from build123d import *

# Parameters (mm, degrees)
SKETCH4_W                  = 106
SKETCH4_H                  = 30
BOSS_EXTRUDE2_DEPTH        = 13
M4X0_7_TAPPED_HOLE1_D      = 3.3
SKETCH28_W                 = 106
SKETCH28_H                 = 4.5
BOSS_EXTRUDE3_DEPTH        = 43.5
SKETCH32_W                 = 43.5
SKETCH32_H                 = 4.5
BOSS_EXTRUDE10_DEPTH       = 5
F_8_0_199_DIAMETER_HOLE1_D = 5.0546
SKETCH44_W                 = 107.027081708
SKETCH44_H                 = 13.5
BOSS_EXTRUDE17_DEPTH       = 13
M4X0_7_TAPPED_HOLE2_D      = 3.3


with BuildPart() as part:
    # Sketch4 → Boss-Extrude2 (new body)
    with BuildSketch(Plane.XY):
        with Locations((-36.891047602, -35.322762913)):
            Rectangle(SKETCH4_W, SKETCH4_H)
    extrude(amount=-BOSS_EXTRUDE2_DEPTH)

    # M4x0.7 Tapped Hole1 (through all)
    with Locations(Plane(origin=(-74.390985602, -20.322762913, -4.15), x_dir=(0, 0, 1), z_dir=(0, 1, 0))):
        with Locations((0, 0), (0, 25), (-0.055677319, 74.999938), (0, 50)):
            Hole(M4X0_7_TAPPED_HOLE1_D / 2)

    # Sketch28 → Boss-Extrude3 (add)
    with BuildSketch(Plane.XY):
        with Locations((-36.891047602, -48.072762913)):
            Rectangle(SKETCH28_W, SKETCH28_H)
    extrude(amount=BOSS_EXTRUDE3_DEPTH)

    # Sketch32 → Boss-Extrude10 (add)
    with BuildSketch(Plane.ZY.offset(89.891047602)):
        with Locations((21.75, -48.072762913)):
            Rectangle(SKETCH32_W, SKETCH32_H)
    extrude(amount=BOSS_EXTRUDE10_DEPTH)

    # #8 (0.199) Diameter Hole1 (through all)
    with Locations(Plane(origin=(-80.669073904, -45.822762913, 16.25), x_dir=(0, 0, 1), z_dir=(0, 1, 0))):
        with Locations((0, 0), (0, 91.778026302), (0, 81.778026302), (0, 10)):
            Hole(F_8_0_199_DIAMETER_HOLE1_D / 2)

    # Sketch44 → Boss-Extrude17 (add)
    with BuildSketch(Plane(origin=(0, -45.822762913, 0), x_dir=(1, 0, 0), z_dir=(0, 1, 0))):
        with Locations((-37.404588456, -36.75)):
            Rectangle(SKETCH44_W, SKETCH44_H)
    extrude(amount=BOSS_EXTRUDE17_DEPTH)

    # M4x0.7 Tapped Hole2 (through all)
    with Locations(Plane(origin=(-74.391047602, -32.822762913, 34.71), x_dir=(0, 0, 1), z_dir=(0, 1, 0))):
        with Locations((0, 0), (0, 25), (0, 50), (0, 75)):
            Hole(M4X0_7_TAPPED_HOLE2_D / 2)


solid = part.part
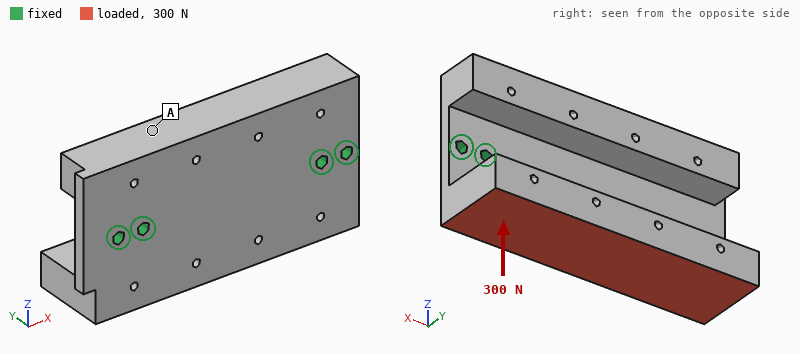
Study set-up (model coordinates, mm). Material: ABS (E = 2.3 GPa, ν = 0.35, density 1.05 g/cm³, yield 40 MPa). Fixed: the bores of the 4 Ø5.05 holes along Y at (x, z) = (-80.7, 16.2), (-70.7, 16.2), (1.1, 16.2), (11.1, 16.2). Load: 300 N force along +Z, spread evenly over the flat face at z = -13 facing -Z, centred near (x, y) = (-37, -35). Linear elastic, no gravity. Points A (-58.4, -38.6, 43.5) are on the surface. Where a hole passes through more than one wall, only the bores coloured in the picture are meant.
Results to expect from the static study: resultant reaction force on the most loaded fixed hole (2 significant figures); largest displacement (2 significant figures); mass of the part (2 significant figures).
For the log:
130 N
1.3 mm
84 g
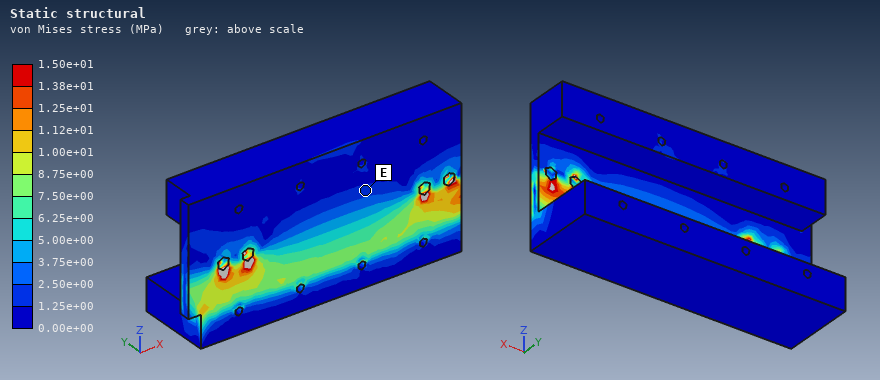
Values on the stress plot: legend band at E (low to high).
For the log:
1.25e+00 to 2.50e+00 MPa
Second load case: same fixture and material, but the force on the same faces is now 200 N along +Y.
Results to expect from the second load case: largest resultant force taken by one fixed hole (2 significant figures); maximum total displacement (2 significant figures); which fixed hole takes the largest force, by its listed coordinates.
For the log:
78 N
1.4 mm
(1.1, 16.2)
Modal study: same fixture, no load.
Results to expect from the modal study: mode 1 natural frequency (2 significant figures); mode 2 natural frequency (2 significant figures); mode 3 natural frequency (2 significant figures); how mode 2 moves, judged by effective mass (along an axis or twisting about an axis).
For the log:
360 Hz
650 Hz
1000 Hz
along Y
